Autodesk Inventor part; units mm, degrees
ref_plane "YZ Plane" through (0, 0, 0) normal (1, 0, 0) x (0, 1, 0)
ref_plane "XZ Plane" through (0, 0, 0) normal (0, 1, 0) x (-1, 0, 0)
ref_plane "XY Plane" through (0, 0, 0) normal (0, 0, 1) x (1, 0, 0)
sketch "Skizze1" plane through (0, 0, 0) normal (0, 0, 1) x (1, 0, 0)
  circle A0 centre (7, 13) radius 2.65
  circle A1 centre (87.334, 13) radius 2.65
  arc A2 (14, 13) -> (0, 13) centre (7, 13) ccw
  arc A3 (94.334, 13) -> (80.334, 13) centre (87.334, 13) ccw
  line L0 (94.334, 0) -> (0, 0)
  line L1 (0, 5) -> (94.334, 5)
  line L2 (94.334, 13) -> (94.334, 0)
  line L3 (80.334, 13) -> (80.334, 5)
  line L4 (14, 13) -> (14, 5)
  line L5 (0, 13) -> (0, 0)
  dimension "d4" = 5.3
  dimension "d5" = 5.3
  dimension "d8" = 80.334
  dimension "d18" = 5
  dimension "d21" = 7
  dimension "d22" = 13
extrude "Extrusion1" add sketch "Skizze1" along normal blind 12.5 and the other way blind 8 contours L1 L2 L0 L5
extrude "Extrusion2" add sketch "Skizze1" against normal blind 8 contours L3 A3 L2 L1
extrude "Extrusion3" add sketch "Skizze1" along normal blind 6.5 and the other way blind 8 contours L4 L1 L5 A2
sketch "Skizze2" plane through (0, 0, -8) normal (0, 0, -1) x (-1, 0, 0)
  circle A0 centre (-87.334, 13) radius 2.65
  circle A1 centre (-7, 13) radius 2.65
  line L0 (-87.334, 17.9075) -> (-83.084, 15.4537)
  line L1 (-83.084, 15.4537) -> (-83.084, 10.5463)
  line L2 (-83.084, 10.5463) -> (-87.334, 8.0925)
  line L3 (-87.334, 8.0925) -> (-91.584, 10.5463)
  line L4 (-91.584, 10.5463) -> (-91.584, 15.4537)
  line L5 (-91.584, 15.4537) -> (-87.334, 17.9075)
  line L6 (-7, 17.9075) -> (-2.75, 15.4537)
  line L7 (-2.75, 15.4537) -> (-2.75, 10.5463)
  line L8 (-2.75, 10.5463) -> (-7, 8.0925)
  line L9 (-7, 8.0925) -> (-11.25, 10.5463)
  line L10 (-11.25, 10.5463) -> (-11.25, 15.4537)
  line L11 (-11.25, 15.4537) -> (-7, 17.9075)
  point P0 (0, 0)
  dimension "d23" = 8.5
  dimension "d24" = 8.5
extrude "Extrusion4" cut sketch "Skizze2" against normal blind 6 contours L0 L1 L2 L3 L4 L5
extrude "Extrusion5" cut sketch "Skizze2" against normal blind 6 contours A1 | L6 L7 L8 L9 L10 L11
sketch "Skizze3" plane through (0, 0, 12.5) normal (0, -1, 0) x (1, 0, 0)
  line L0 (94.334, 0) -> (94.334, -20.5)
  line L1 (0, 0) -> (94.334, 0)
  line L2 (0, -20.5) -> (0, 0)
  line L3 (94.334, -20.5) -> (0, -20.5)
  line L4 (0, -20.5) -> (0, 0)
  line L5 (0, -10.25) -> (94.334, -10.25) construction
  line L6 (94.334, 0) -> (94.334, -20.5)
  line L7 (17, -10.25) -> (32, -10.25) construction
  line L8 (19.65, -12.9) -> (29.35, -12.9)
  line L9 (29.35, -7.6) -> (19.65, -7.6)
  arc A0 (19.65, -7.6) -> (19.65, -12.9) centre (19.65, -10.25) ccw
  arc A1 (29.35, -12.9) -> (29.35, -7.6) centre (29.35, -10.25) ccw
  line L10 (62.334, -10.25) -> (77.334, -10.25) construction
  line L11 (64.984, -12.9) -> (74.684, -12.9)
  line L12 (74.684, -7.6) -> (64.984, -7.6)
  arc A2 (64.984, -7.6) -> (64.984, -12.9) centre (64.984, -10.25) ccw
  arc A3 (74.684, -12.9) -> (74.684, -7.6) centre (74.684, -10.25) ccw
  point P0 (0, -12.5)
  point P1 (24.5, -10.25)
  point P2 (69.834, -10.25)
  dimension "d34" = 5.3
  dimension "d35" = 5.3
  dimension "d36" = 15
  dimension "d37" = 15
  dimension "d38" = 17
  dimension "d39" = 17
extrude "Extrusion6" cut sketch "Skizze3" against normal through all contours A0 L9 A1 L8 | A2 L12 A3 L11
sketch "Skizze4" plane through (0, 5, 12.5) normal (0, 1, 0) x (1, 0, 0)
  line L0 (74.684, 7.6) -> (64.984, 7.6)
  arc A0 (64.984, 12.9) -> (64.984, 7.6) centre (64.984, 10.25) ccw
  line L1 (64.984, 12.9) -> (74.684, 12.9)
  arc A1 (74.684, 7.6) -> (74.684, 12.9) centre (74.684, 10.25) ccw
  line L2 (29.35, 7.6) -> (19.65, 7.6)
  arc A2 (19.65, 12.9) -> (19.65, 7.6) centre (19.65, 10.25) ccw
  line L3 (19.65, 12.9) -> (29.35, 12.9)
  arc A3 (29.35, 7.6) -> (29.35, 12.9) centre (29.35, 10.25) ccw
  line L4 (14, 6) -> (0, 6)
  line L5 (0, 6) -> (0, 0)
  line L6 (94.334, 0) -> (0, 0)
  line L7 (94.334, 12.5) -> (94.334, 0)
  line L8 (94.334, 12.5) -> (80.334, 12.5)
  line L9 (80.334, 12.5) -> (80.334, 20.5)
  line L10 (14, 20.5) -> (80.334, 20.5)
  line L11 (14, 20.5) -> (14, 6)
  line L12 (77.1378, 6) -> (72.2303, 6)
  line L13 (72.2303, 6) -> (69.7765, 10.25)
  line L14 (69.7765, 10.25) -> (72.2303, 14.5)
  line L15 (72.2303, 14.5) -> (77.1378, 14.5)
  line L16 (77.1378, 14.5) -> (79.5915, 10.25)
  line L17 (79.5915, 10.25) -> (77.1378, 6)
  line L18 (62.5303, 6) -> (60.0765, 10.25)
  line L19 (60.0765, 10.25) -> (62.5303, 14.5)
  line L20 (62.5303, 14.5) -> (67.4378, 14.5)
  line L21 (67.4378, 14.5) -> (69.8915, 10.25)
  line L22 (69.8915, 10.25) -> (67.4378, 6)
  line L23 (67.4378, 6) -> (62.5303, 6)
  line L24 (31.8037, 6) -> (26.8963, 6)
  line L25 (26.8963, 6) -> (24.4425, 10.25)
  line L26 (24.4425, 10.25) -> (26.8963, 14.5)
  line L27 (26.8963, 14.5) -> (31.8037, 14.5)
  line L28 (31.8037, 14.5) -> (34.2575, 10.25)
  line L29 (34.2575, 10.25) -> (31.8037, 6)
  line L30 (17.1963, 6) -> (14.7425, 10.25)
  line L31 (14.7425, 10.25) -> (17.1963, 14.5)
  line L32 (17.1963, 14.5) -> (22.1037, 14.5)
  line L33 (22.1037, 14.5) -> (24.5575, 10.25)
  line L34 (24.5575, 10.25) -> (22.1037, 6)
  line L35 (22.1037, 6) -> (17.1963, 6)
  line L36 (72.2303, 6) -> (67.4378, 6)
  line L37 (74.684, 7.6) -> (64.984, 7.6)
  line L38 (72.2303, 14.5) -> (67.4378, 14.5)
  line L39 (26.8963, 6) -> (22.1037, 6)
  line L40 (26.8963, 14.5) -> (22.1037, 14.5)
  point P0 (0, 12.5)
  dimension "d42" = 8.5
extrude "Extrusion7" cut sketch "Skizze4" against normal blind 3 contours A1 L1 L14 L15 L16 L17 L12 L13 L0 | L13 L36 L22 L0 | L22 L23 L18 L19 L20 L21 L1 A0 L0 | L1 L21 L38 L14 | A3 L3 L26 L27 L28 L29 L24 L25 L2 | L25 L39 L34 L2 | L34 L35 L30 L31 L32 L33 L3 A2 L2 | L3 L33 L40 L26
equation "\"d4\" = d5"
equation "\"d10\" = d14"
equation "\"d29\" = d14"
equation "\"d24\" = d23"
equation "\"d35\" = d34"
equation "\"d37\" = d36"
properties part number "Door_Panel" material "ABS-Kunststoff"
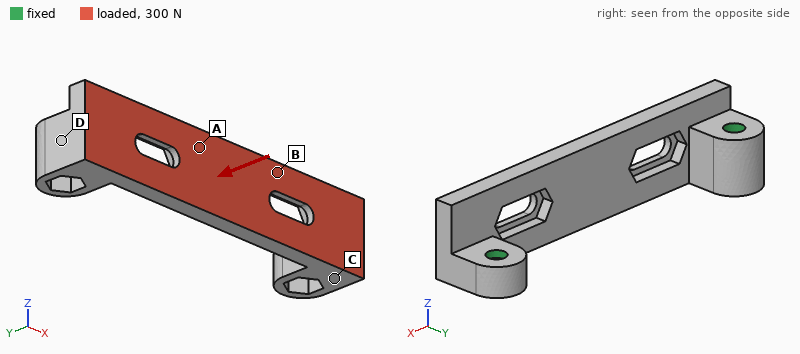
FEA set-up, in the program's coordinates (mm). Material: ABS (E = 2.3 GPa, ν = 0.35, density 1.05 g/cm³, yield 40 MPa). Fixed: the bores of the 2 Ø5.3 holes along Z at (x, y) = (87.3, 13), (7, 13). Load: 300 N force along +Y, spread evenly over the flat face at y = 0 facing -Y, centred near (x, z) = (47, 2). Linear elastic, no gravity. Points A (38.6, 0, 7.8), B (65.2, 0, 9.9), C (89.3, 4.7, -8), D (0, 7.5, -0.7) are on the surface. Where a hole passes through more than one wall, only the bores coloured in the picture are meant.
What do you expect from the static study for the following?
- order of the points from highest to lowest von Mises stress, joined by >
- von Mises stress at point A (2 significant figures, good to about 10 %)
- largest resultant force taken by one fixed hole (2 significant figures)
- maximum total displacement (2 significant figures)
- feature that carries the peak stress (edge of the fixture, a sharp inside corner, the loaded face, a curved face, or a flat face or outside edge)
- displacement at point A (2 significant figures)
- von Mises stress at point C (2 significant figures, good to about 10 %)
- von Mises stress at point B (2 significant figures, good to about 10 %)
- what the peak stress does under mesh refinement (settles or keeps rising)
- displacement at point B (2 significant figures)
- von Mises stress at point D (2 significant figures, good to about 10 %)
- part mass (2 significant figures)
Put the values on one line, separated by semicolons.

A > B > C > D; 9.5 MPa; 180 N; 0.89 mm; edge of the fixture; 0.71 mm; 3.9 MPa; 6.5 MPa; keeps rising; 0.68 mm; 1.6 MPa; 12 g
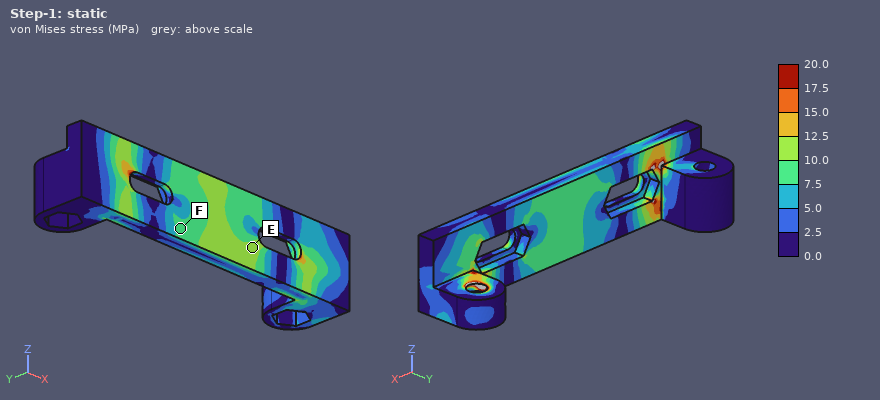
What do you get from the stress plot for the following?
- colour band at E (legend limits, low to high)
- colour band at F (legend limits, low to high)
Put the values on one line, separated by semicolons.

10.0 to 12.5 MPa; 7.5 to 10.0 MPa
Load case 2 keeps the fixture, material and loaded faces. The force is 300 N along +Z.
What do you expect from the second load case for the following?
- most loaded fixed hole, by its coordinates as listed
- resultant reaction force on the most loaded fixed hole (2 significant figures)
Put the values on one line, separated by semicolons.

(7, 13); 170 N
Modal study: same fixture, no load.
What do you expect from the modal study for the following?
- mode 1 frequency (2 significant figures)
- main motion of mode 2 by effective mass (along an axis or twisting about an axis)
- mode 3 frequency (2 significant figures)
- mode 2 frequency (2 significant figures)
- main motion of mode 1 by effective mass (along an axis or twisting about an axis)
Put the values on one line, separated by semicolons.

1200 Hz; along Z; 2100 Hz; 1500 Hz; along Y
